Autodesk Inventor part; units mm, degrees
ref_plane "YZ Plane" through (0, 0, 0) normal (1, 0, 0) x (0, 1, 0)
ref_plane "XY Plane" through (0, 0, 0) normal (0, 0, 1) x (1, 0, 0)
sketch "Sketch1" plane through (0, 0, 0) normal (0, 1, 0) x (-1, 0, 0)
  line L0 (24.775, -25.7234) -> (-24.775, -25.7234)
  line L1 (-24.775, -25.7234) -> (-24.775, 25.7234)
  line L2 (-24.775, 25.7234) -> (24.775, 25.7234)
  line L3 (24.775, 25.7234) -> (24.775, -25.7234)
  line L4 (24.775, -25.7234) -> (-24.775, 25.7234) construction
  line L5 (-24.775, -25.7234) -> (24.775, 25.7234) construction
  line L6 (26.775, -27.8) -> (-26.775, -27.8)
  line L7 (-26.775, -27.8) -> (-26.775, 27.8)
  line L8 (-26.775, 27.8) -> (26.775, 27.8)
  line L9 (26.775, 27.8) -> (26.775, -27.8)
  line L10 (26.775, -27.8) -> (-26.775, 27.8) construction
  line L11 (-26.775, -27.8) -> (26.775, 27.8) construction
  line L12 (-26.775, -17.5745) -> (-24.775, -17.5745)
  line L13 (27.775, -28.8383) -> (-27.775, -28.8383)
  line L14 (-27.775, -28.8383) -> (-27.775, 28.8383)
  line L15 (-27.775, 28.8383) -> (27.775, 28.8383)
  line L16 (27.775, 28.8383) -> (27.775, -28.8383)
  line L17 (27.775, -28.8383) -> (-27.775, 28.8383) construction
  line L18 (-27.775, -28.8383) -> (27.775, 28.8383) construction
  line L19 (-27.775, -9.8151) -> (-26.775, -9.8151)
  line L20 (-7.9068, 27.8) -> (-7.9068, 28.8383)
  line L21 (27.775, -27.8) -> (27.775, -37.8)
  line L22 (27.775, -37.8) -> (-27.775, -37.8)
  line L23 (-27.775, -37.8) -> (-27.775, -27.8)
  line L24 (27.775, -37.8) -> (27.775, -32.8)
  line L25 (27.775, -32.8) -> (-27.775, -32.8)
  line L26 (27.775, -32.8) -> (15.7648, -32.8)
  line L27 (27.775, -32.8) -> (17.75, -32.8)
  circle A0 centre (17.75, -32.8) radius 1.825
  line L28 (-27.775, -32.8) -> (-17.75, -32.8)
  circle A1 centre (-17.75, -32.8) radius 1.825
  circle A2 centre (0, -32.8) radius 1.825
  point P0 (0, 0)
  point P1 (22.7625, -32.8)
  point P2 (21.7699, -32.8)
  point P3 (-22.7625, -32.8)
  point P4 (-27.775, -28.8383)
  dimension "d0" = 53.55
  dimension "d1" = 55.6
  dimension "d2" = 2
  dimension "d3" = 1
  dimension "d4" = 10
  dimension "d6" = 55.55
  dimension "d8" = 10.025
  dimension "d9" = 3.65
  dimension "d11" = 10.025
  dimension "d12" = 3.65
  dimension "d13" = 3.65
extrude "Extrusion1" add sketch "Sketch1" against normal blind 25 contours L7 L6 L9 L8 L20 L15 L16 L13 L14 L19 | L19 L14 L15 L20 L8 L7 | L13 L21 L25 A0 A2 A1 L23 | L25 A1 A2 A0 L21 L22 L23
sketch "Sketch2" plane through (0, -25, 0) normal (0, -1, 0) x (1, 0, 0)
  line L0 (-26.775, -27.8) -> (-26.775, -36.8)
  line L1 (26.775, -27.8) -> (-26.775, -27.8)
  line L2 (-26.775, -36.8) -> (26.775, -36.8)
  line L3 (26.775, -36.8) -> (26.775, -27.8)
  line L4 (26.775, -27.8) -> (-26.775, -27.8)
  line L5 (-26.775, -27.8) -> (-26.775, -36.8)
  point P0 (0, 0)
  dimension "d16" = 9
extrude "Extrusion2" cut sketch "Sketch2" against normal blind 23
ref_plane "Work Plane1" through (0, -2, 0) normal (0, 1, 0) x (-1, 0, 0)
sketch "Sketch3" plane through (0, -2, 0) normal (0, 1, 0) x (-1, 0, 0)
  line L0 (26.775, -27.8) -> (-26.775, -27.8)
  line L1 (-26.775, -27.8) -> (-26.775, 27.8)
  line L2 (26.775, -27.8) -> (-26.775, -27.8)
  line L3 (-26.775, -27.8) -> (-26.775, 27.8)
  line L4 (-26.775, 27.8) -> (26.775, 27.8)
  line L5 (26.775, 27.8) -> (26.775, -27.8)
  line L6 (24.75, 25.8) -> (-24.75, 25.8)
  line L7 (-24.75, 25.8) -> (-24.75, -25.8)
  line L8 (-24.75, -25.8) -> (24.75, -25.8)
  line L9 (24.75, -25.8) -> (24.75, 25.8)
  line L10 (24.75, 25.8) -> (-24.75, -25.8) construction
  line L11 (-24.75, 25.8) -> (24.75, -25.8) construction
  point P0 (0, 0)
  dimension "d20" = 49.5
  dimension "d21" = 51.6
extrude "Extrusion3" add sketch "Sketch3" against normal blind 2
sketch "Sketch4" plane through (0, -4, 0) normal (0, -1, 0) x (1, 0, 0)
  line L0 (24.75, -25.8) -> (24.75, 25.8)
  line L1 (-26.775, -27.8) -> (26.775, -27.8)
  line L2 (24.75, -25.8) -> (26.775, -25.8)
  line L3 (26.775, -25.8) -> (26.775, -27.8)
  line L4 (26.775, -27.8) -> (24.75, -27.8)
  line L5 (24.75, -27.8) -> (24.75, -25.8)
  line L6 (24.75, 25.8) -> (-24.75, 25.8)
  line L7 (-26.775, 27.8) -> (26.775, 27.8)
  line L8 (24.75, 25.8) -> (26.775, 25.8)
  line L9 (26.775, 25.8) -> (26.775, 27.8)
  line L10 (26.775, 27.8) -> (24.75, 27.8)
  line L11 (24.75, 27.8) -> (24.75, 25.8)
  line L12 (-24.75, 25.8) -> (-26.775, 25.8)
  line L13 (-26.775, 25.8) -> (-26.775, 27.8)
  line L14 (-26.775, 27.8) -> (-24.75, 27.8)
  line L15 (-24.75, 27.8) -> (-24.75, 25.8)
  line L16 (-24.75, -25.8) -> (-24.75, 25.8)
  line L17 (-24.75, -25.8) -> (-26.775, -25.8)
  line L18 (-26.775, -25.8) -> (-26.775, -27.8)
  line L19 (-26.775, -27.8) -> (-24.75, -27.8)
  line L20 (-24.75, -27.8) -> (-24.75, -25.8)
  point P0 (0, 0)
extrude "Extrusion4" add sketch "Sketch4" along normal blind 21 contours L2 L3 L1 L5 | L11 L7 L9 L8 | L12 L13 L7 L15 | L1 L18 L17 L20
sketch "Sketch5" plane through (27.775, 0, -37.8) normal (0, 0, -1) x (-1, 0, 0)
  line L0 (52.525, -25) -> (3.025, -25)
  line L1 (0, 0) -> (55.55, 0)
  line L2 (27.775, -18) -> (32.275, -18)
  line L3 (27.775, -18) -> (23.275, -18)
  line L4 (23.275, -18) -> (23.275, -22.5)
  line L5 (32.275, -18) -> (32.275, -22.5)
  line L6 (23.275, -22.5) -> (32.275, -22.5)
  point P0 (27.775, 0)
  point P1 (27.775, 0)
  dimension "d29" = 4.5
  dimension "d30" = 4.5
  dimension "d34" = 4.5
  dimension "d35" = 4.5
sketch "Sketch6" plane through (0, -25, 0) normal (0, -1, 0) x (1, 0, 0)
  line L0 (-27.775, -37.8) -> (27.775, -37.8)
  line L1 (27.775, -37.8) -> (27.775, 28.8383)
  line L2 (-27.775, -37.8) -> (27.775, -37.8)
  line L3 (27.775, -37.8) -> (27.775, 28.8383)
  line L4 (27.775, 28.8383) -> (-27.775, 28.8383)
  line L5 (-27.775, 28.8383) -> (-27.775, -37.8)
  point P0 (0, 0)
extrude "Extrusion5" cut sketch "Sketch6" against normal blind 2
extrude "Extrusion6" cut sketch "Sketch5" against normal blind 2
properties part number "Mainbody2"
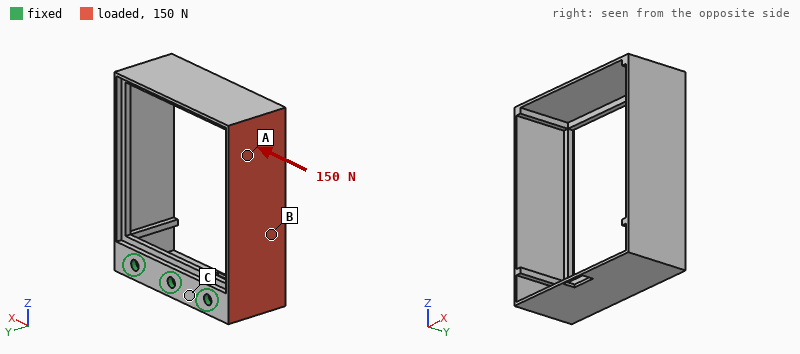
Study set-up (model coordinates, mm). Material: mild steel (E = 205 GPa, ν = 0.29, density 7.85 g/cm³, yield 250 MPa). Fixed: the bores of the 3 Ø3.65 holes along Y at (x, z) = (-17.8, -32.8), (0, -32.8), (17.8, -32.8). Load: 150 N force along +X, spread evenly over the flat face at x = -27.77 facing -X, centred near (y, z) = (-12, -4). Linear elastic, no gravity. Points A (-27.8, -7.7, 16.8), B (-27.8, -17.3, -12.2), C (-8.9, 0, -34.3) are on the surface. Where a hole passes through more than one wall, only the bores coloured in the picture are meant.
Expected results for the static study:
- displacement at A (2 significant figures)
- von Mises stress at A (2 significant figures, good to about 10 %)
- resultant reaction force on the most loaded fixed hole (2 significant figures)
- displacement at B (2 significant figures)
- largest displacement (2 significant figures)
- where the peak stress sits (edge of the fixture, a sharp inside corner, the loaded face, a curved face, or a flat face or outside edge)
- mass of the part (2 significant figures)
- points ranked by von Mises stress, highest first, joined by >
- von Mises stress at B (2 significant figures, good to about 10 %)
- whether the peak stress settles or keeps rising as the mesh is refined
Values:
0.33 mm
54 MPa
110 N
0.17 mm
0.40 mm
a sharp inside corner
60 g
A > B > C
31 MPa
keeps rising
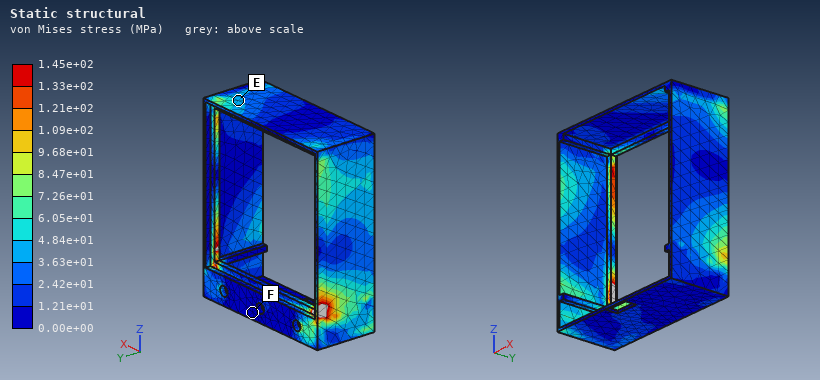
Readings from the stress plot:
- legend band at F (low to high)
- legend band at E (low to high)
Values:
0.00e+00 to 1.21e+01 MPa
3.63e+01 to 4.84e+01 MPa
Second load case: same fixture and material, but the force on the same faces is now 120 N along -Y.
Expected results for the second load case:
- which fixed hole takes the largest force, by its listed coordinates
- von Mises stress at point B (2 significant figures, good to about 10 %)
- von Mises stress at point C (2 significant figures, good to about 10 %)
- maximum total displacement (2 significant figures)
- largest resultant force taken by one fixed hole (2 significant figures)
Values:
(-17.8, -32.8)
26 MPa
25 MPa
0.38 mm
190 N
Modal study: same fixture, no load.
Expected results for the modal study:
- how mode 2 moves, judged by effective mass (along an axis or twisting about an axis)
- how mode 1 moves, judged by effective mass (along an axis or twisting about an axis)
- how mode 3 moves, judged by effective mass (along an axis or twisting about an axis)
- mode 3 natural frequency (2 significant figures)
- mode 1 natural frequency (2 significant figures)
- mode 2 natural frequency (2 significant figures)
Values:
along Y
along X
twisting about Z
770 Hz
460 Hz
590 Hz
